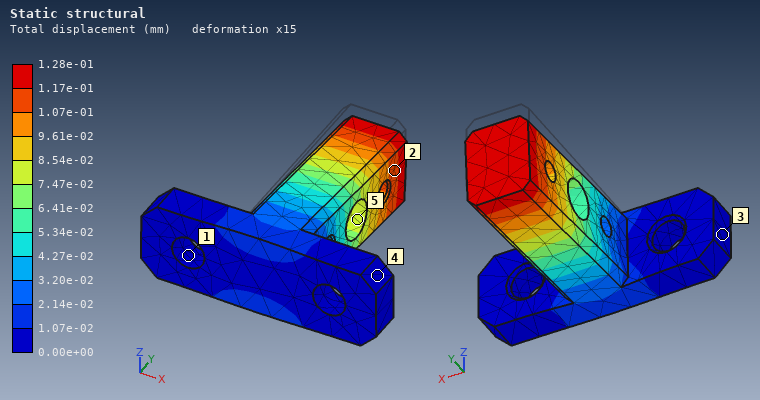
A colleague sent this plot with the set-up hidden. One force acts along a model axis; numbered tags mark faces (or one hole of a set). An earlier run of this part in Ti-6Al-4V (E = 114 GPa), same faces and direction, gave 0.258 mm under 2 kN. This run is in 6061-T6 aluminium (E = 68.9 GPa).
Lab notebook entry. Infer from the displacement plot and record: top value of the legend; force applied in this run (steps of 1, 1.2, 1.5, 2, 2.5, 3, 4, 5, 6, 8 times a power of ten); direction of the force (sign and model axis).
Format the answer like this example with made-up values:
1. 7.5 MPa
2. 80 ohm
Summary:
1. 1.28e-01 mm
2. 600 N
3. -Z
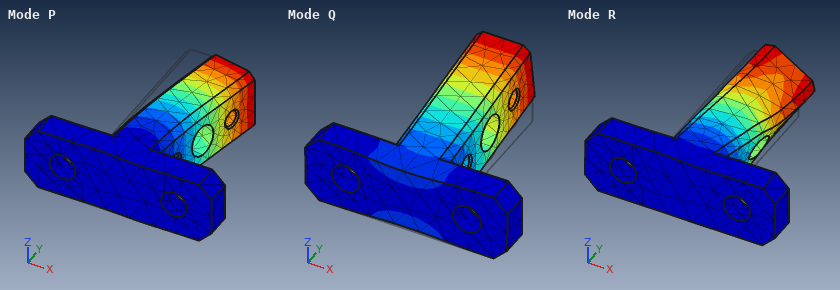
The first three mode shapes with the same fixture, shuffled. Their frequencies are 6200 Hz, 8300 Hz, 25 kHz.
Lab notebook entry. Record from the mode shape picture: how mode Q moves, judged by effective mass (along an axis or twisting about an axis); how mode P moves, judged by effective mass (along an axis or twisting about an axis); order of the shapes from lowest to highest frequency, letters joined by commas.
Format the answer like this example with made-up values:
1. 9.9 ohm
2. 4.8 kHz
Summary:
1. along Z
2. along X
3. Q, P, R
